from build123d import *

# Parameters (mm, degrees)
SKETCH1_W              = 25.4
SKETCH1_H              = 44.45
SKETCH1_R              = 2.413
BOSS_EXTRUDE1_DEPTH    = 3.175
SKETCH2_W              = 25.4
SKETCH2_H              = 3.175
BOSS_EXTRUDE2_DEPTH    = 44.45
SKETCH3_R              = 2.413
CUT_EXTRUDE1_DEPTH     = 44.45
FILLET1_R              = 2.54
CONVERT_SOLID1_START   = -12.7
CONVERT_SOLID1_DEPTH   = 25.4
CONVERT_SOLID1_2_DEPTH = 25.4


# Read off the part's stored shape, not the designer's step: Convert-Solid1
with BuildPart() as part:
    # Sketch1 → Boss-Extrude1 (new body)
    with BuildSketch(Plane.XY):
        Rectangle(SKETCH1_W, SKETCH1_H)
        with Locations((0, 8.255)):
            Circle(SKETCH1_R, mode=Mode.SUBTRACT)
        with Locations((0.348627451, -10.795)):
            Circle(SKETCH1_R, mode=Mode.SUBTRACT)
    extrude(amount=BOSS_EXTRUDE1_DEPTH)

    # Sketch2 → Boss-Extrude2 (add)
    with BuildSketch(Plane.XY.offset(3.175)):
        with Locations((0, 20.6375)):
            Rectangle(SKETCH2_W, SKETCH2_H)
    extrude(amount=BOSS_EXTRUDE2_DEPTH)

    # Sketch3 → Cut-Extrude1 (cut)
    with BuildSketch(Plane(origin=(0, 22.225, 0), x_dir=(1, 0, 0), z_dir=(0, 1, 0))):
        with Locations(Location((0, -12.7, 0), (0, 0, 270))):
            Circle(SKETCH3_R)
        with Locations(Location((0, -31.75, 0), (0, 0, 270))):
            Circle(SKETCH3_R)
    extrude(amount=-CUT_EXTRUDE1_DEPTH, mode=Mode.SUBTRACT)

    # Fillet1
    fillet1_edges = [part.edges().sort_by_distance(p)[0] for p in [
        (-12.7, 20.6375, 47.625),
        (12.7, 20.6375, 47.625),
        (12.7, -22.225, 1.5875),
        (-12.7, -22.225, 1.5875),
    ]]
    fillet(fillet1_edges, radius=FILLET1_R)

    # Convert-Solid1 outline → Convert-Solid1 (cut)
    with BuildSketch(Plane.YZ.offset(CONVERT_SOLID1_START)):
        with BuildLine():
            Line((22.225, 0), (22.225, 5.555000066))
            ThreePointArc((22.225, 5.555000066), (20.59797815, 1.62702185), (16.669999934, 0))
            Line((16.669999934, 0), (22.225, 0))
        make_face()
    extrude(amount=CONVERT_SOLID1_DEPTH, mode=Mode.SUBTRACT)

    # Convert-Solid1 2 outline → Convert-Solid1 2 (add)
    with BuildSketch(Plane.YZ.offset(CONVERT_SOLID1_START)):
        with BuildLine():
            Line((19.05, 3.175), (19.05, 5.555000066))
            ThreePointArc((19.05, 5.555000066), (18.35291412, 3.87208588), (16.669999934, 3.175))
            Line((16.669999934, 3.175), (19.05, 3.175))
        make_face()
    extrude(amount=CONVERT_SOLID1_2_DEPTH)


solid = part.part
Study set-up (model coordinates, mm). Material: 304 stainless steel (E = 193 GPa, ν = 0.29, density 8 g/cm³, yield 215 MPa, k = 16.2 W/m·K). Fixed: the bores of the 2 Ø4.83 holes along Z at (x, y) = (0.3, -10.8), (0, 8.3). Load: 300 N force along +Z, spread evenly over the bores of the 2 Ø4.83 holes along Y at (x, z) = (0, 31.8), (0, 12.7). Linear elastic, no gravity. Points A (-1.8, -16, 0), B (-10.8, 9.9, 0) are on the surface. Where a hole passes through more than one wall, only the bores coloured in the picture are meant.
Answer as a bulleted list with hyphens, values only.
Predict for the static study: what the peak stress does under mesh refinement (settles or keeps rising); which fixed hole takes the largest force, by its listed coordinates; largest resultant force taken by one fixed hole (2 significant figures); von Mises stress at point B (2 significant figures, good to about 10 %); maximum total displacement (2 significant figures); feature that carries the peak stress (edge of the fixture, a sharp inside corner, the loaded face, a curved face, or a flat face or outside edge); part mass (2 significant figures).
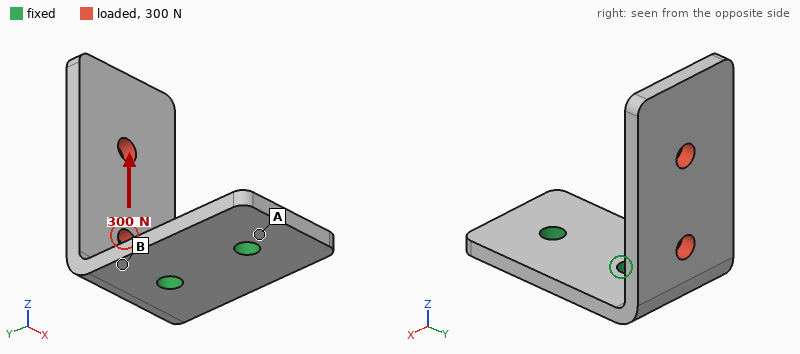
- keeps rising
- (0, 8.3)
- 340 N
- 34 MPa
- 79 µm
- edge of the fixture
- 54 g
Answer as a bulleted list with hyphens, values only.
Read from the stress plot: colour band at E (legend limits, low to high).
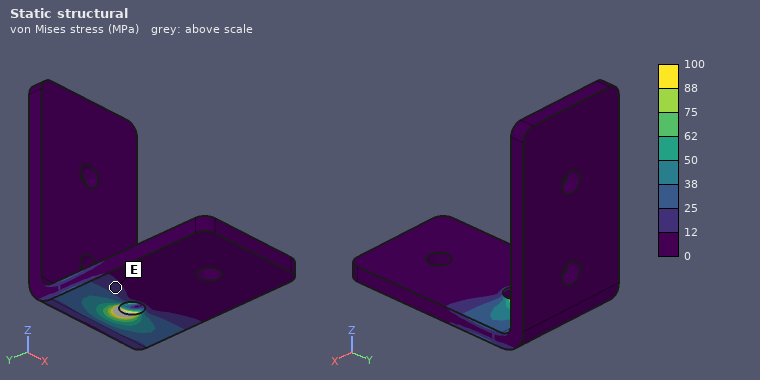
- 12 to 25 MPa
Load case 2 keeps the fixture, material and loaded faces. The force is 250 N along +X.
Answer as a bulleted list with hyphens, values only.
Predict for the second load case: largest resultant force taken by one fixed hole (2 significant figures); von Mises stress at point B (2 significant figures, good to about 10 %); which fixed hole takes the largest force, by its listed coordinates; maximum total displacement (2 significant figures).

- 360 N
- 50 MPa
- (0, 8.3)
- 0.12 mm
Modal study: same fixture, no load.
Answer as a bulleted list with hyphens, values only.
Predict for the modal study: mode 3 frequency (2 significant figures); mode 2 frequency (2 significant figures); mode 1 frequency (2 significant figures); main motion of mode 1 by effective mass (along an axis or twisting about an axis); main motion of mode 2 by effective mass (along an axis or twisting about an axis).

- 4300 Hz
- 1500 Hz
- 860 Hz
- along Y
- along X
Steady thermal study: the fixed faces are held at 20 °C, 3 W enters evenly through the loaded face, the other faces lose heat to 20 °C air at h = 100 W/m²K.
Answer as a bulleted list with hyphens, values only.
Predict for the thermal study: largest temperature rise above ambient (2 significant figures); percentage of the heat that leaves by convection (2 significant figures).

- 16 K
- 86 %
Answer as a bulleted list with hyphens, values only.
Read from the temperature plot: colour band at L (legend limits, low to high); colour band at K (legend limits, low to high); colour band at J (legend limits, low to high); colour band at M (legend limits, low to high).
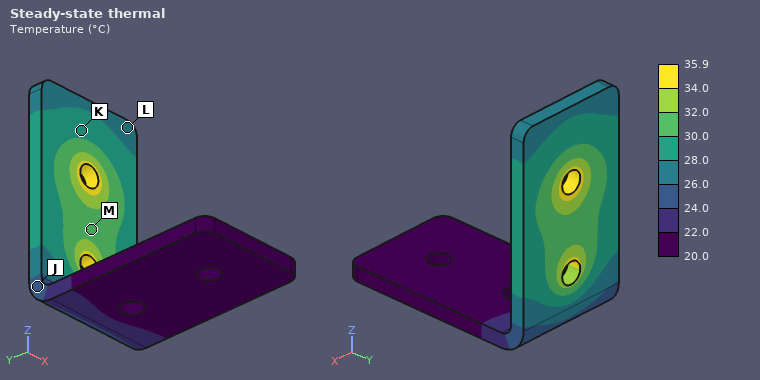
- 26.0 to 28.0 °C
- 28.0 to 30.0 °C
- 24.0 to 26.0 °C
- 30.0 to 32.0 °C
